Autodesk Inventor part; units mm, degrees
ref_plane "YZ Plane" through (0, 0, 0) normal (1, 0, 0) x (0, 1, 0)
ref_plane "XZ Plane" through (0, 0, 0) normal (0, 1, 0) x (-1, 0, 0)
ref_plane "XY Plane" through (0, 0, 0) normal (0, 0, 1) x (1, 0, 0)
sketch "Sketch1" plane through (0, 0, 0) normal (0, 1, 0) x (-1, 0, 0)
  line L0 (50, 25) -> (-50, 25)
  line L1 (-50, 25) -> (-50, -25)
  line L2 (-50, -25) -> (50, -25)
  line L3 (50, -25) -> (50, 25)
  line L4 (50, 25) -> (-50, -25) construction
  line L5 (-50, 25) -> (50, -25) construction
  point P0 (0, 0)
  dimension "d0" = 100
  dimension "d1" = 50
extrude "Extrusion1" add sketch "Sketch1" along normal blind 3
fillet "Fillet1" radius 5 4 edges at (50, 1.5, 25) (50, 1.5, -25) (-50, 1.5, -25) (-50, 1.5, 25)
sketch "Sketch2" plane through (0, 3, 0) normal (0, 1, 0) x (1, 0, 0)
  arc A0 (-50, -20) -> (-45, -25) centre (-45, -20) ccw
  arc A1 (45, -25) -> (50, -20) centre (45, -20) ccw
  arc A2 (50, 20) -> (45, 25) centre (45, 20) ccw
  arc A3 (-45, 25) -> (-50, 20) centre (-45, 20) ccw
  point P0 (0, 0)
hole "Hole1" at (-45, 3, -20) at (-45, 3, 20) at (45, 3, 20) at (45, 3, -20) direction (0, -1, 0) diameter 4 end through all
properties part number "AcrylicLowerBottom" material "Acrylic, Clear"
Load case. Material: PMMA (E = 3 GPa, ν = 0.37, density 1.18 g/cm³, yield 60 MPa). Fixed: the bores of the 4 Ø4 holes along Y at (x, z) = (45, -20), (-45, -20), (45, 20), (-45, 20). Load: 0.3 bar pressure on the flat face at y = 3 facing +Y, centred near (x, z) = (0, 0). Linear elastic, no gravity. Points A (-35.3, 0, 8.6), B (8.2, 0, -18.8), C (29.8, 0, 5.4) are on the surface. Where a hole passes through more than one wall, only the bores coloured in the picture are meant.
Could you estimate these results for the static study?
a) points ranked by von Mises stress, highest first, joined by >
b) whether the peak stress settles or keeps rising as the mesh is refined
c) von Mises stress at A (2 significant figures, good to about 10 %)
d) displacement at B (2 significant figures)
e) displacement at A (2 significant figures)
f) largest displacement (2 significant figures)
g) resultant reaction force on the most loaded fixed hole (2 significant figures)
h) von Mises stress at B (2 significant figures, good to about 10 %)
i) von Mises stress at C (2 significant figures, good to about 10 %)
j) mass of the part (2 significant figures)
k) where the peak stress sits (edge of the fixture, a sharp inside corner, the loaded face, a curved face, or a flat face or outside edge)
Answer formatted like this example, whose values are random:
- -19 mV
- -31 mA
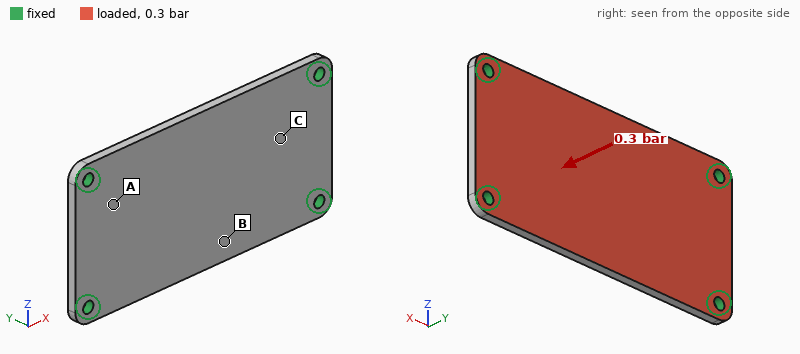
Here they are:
- B > A > C
- keeps rising
- 3.8 MPa
- 0.82 mm
- 0.20 mm
- 0.91 mm
- 37 N
- 6.7 MPa
- 2.1 MPa
- 17 g
- edge of the fixture
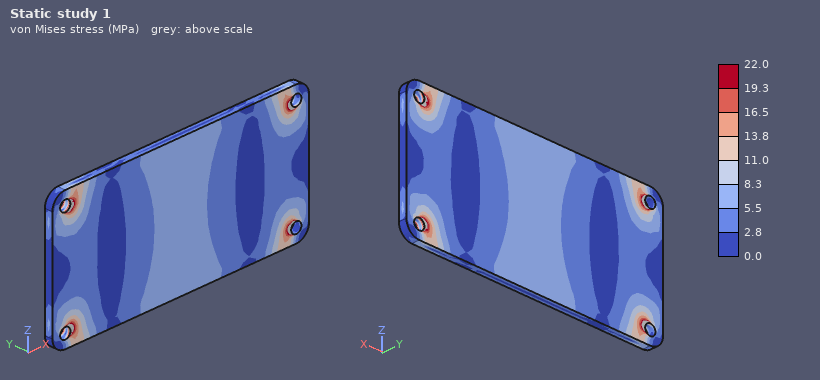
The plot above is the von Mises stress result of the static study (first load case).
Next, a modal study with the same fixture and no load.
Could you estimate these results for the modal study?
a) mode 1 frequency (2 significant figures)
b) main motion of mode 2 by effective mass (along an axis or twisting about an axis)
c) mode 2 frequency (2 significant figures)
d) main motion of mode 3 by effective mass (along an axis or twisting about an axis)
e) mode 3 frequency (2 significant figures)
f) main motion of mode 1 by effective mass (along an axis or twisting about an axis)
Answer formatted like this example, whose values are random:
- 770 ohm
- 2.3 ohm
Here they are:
- 560 Hz
- twisting about X
- 950 Hz
- twisting about Z
- 1600 Hz
- along Y
